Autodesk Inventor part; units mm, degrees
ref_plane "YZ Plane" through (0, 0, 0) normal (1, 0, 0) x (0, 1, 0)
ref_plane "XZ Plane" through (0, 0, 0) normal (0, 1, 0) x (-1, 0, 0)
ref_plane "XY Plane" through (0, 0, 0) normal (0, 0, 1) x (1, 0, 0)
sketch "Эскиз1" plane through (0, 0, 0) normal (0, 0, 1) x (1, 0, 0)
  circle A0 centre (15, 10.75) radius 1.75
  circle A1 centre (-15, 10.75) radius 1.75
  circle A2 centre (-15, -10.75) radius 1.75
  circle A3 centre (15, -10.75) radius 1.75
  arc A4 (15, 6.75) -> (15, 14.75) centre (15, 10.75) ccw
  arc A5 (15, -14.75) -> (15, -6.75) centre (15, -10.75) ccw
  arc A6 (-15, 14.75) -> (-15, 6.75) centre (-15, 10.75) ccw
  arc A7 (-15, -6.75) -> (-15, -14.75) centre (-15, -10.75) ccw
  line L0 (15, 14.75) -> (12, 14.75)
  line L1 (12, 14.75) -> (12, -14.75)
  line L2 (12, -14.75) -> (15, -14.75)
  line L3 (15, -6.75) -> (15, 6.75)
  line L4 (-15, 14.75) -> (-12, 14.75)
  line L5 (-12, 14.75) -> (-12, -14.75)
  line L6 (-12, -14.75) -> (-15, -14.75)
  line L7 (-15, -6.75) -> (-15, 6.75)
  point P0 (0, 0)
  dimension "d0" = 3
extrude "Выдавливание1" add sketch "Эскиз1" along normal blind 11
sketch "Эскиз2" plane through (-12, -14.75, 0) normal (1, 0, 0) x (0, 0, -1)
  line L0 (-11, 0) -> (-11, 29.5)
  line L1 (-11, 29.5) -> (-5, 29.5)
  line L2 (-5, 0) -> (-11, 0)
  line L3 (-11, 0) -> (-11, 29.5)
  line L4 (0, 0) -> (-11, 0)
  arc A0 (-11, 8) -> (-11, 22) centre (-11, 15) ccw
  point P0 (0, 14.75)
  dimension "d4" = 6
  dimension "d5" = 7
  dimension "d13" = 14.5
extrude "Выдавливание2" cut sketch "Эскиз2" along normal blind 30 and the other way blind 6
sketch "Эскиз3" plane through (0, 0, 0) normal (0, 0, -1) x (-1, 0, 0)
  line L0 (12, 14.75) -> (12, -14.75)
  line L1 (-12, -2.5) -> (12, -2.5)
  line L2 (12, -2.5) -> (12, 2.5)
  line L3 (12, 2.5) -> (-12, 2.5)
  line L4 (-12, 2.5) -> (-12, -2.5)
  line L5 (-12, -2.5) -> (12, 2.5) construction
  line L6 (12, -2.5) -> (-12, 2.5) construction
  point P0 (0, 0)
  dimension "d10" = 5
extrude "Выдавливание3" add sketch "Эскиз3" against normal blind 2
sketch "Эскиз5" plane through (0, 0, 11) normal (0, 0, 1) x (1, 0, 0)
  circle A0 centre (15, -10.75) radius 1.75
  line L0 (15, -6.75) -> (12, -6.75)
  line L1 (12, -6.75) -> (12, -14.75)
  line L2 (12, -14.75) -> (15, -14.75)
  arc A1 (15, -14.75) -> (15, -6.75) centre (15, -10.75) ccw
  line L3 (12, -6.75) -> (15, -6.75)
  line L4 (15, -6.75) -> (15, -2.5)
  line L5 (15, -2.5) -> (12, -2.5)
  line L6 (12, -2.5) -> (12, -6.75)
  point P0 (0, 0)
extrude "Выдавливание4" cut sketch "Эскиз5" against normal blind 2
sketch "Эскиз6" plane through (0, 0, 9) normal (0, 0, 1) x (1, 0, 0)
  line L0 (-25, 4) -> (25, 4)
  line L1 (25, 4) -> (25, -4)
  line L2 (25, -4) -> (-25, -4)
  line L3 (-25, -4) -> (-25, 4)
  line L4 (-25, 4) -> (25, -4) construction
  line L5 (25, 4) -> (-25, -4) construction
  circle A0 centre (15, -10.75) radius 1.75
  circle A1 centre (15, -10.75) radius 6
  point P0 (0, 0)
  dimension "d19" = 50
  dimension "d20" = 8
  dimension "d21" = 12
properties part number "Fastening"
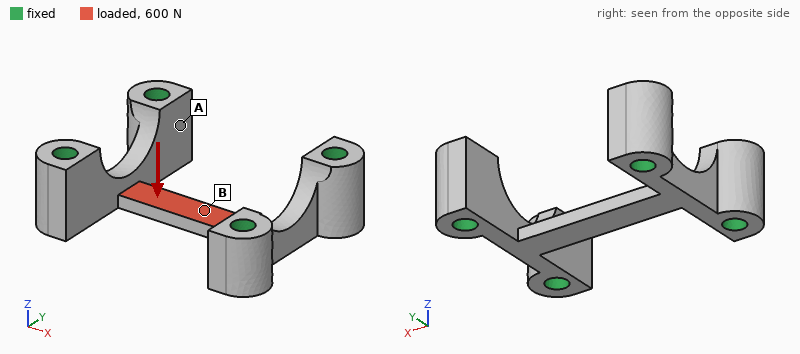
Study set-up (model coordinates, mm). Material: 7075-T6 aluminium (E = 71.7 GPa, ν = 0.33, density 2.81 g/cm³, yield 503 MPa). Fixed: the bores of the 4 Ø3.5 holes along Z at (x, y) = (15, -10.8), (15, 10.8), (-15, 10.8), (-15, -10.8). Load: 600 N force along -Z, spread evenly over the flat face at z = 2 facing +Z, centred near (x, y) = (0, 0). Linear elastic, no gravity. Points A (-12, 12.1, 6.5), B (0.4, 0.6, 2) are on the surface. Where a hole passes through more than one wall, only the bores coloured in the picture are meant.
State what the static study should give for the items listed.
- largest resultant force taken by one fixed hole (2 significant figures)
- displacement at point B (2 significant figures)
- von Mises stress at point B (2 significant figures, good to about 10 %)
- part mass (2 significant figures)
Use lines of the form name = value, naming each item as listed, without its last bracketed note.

largest resultant force taken by one fixed hole = 210 N
displacement at point B = 0.15 mm
von Mises stress at point B = 200 MPa
part mass = 6.5 g
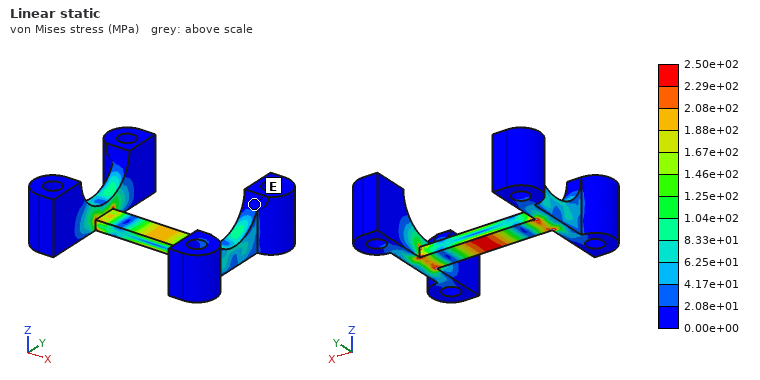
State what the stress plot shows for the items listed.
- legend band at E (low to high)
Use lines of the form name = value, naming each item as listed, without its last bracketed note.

legend band at E = 0.00e+00 to 2.08e+01 MPa
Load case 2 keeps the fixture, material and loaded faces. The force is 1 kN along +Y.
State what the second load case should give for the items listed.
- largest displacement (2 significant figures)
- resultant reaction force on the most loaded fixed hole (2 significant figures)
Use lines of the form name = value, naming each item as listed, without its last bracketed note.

largest displacement = 80 µm
resultant reaction force on the most loaded fixed hole = 330 N
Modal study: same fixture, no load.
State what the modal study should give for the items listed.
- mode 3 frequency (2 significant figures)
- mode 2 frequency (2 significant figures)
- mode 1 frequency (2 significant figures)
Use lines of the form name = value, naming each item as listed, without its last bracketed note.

mode 3 frequency = 32 kHz
mode 2 frequency = 28 kHz
mode 1 frequency = 14 kHz
